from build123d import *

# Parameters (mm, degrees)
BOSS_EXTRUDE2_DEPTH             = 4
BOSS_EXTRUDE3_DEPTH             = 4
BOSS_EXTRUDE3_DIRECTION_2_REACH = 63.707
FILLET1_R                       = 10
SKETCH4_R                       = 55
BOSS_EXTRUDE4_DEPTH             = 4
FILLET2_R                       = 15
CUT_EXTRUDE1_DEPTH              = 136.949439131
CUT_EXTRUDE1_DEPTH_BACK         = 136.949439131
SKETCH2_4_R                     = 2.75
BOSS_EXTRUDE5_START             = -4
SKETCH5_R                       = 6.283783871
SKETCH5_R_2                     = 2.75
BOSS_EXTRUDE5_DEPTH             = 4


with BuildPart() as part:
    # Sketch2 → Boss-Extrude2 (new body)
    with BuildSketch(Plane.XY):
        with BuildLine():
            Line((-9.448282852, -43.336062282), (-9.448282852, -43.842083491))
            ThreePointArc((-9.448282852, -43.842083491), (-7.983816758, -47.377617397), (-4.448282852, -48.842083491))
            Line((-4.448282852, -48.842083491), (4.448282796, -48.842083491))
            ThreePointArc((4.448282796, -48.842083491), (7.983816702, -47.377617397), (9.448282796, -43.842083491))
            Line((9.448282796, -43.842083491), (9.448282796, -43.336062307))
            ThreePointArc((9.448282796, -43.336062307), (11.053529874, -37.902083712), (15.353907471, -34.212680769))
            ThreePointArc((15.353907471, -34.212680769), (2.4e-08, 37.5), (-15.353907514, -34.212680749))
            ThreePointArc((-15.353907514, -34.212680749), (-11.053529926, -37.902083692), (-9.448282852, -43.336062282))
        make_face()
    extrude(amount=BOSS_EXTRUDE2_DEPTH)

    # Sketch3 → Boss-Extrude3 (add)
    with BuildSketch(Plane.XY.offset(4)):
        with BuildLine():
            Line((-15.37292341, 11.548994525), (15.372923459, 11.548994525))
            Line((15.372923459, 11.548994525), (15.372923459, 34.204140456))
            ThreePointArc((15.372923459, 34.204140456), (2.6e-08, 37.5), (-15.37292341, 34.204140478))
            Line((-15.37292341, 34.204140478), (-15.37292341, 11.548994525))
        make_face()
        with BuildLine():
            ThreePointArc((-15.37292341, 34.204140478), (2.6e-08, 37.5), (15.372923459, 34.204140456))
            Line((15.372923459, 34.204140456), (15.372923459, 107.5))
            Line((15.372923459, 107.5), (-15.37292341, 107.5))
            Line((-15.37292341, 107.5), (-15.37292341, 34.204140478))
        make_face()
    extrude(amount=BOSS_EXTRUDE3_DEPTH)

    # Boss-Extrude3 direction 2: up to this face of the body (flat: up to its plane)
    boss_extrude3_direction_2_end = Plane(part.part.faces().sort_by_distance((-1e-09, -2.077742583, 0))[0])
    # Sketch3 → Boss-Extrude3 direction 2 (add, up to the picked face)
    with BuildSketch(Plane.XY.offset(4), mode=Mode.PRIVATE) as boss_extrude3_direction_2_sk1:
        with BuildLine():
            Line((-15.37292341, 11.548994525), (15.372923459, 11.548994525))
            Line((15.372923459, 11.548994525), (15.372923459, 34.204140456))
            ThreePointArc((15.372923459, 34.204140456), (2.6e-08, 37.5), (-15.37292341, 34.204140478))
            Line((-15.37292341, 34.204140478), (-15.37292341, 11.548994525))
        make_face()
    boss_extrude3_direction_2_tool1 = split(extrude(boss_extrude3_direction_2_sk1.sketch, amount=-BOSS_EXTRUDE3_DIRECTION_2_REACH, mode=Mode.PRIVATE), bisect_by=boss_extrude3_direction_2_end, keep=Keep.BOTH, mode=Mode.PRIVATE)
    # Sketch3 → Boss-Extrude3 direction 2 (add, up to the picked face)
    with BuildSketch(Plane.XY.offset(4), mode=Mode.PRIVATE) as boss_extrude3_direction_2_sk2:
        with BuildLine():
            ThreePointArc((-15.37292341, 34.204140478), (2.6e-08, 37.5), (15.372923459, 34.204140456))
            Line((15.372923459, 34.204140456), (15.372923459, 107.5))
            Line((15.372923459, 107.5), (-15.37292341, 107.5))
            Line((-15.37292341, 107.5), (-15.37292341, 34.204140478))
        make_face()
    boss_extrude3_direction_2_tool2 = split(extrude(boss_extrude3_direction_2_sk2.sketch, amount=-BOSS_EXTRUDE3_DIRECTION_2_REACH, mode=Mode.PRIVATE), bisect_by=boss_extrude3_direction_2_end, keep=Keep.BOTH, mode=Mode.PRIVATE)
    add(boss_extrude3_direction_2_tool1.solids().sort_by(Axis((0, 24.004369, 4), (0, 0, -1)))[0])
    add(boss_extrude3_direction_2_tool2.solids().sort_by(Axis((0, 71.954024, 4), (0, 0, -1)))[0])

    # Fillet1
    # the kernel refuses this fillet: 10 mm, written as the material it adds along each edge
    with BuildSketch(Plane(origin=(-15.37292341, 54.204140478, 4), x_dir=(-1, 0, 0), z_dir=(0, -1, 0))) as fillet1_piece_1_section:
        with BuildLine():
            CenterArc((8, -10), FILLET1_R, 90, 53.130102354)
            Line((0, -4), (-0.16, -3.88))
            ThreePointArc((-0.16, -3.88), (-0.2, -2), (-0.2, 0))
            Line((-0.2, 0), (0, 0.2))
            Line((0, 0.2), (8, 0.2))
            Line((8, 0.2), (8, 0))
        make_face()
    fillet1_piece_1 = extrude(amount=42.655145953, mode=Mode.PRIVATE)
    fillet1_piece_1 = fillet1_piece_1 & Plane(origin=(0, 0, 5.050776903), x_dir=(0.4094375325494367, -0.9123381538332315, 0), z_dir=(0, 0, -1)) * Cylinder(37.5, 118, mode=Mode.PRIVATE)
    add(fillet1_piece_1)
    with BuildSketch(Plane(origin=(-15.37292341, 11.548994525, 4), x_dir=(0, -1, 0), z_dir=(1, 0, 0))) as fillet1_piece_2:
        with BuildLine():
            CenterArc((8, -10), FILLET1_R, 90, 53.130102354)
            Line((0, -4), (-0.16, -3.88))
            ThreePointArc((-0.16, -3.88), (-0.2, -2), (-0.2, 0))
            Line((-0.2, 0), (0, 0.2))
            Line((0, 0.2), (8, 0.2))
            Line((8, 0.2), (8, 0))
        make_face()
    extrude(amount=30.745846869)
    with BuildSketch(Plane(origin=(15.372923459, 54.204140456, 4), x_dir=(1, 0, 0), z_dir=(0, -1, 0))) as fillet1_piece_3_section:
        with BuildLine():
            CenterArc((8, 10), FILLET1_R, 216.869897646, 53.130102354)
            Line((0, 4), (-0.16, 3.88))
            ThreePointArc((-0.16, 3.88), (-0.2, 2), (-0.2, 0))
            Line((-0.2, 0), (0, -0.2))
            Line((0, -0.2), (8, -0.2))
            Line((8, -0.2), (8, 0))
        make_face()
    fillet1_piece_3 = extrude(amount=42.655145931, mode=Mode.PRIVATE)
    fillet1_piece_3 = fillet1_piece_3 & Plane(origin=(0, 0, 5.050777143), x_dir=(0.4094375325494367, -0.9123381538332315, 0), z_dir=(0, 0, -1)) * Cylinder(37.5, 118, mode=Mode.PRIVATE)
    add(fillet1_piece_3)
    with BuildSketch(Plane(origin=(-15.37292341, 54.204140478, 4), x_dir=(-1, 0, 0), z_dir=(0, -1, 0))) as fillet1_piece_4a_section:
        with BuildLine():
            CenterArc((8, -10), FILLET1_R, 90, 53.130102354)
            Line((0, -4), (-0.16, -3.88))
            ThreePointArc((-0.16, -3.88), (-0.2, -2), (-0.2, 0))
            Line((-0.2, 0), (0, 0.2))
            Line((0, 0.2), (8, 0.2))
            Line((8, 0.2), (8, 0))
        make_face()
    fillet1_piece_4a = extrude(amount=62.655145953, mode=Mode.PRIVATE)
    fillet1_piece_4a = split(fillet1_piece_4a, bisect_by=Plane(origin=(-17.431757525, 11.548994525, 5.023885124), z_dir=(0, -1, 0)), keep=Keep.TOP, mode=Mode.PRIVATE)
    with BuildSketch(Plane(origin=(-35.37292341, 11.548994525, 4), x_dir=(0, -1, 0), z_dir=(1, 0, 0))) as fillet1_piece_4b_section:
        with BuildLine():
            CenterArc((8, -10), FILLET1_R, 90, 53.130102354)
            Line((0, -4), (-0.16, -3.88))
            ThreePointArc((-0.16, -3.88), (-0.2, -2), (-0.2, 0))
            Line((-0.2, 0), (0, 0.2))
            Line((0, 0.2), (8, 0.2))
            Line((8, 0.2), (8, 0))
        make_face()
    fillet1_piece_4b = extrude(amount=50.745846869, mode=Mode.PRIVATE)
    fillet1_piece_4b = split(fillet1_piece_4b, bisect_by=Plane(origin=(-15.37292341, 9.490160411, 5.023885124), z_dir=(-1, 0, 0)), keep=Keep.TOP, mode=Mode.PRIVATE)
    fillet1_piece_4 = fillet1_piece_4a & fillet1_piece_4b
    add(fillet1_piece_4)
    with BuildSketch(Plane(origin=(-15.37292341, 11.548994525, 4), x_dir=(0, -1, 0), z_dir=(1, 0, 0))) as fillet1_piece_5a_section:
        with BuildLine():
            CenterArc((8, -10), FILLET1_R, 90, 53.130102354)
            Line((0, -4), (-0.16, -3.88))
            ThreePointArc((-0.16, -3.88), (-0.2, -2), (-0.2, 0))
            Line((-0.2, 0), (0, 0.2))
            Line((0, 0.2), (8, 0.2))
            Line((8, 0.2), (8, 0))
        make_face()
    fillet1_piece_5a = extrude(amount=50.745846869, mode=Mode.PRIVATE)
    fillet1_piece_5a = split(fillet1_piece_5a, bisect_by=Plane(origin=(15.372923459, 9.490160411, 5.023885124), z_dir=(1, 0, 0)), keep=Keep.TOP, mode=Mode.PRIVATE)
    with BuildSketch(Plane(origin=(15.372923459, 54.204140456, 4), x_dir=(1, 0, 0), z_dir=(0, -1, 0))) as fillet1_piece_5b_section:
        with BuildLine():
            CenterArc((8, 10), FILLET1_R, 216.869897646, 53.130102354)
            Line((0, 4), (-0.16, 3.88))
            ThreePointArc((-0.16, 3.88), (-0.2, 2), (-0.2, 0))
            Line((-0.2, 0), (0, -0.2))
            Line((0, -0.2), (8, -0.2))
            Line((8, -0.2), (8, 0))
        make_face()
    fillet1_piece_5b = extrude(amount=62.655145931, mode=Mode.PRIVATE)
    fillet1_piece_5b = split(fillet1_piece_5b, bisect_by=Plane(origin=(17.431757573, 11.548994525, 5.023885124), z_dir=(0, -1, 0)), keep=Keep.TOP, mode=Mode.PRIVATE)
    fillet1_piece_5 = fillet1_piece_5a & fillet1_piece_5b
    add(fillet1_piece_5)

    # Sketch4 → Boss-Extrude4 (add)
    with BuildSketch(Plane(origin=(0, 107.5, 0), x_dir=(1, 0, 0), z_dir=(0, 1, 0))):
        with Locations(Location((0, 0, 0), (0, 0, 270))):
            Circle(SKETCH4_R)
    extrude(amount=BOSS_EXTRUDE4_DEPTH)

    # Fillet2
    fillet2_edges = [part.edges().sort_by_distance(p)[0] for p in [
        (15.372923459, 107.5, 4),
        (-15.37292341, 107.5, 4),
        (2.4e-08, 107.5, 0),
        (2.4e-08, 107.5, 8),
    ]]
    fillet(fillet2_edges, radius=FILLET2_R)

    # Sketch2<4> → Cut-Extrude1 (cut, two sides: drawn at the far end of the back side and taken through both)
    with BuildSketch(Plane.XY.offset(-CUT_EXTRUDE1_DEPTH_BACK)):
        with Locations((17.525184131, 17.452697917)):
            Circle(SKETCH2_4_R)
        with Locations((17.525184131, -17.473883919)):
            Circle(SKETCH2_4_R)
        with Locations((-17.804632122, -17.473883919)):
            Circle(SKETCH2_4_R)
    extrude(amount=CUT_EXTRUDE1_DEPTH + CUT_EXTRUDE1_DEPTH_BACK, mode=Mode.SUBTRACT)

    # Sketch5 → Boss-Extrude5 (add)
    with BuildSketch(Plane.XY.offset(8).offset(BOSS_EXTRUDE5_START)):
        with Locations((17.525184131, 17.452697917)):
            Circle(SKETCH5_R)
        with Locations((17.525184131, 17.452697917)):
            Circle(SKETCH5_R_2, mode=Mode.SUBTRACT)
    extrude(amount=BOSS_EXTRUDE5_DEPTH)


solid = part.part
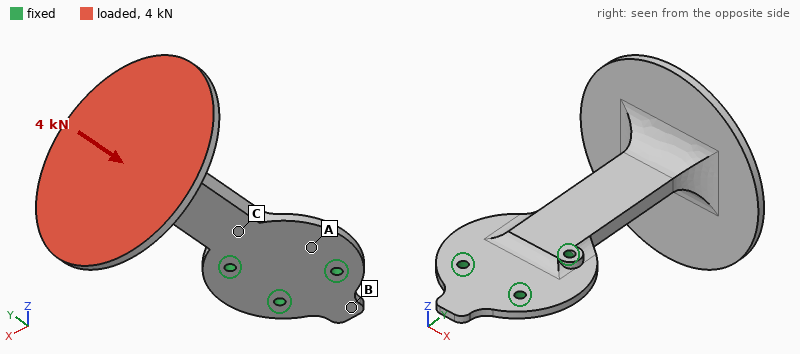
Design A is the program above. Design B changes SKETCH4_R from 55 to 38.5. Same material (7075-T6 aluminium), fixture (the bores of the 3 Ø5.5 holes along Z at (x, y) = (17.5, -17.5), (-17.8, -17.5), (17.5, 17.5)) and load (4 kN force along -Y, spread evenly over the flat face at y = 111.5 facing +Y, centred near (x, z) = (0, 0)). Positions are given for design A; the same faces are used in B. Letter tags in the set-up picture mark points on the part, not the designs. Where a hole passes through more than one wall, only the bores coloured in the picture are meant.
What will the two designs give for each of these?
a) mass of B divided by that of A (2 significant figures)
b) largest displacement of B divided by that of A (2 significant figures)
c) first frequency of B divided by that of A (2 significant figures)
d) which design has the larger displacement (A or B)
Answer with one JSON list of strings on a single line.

["0.77", "0.72", "1.4", "A"]
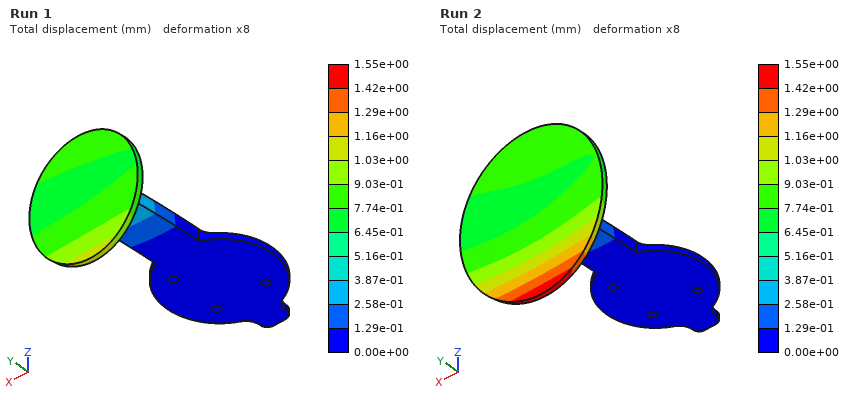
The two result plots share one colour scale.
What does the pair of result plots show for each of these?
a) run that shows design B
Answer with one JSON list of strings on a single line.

["Run 1"]
